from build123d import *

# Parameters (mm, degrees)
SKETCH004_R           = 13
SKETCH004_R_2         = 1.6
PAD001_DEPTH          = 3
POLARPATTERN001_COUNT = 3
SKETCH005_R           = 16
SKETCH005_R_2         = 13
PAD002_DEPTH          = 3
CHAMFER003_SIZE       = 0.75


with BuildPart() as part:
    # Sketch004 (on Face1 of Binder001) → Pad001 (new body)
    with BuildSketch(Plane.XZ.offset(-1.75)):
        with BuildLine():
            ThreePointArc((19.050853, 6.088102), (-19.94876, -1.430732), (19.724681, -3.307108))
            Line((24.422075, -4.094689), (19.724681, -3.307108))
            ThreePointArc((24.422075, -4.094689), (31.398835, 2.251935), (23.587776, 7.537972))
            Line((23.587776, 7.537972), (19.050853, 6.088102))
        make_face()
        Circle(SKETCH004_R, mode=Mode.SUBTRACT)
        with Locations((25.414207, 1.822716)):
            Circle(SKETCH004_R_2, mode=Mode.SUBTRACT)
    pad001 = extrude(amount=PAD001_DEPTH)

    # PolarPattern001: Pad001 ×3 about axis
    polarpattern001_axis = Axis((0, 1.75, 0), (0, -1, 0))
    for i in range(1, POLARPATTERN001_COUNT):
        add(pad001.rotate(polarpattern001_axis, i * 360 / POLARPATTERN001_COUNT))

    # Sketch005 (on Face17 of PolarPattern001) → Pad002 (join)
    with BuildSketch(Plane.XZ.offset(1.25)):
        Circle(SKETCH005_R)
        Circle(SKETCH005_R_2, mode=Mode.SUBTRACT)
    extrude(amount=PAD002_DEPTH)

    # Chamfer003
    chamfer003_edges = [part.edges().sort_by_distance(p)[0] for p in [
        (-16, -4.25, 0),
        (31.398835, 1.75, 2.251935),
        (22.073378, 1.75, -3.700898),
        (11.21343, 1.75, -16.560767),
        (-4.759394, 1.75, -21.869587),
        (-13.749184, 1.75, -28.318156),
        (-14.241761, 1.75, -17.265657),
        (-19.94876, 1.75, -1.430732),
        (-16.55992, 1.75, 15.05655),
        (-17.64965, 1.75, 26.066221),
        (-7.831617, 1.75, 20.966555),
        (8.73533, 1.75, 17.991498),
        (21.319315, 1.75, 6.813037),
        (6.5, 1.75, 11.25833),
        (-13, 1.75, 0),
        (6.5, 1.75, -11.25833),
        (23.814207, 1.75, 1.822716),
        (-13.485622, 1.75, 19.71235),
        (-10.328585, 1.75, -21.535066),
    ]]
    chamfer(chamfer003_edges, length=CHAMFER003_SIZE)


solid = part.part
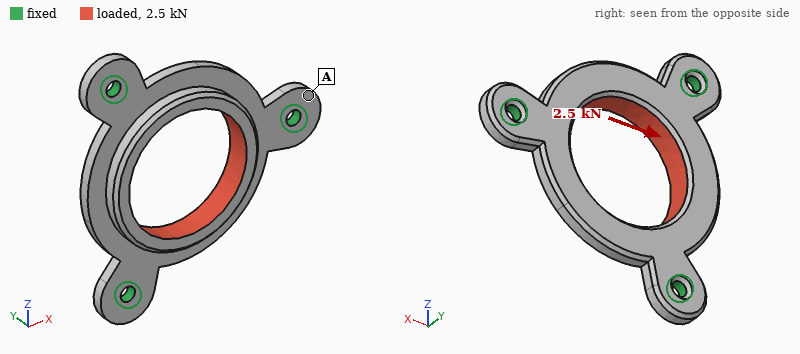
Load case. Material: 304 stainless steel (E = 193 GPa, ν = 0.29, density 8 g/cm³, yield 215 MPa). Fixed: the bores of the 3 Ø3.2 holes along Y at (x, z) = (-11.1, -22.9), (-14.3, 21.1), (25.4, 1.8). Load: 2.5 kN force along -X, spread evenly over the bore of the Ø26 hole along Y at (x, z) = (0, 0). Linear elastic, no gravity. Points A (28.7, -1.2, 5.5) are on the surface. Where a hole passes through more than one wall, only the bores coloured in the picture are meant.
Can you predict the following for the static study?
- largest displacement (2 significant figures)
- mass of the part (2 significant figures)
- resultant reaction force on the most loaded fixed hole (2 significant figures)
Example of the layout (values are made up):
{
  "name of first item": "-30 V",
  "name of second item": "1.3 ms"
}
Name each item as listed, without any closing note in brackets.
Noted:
{
  "largest displacement": "19 µm",
  "mass of the part": "31 g",
  "resultant reaction force on the most loaded fixed hole": "910 N"
}
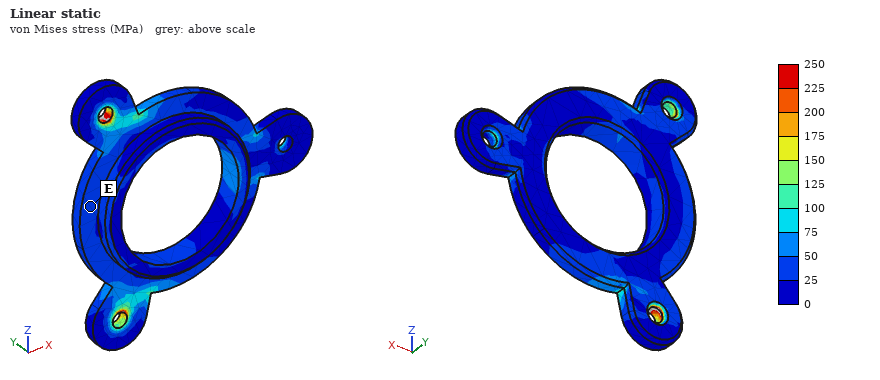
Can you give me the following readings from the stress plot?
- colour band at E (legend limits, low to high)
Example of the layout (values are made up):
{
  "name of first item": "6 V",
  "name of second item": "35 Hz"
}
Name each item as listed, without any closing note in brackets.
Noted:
{
  "colour band at E": "25 to 50 MPa"
}
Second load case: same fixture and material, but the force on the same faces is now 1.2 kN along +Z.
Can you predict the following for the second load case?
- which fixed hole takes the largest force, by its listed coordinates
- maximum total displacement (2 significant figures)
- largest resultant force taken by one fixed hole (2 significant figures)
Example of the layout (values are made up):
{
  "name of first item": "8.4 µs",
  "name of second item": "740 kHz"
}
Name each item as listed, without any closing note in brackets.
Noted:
{
  "which fixed hole takes the largest force, by its listed coordinates": "(25.4, 1.8)",
  "maximum total displacement": "8.2 µm",
  "largest resultant force taken by one fixed hole": "450 N"
}
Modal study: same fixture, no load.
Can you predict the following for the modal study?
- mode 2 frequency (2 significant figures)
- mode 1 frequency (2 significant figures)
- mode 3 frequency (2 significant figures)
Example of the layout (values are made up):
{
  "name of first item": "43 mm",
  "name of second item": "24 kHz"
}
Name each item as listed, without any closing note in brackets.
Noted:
{
  "mode 2 frequency": "8400 Hz",
  "mode 1 frequency": "8300 Hz",
  "mode 3 frequency": "8400 Hz"
}
